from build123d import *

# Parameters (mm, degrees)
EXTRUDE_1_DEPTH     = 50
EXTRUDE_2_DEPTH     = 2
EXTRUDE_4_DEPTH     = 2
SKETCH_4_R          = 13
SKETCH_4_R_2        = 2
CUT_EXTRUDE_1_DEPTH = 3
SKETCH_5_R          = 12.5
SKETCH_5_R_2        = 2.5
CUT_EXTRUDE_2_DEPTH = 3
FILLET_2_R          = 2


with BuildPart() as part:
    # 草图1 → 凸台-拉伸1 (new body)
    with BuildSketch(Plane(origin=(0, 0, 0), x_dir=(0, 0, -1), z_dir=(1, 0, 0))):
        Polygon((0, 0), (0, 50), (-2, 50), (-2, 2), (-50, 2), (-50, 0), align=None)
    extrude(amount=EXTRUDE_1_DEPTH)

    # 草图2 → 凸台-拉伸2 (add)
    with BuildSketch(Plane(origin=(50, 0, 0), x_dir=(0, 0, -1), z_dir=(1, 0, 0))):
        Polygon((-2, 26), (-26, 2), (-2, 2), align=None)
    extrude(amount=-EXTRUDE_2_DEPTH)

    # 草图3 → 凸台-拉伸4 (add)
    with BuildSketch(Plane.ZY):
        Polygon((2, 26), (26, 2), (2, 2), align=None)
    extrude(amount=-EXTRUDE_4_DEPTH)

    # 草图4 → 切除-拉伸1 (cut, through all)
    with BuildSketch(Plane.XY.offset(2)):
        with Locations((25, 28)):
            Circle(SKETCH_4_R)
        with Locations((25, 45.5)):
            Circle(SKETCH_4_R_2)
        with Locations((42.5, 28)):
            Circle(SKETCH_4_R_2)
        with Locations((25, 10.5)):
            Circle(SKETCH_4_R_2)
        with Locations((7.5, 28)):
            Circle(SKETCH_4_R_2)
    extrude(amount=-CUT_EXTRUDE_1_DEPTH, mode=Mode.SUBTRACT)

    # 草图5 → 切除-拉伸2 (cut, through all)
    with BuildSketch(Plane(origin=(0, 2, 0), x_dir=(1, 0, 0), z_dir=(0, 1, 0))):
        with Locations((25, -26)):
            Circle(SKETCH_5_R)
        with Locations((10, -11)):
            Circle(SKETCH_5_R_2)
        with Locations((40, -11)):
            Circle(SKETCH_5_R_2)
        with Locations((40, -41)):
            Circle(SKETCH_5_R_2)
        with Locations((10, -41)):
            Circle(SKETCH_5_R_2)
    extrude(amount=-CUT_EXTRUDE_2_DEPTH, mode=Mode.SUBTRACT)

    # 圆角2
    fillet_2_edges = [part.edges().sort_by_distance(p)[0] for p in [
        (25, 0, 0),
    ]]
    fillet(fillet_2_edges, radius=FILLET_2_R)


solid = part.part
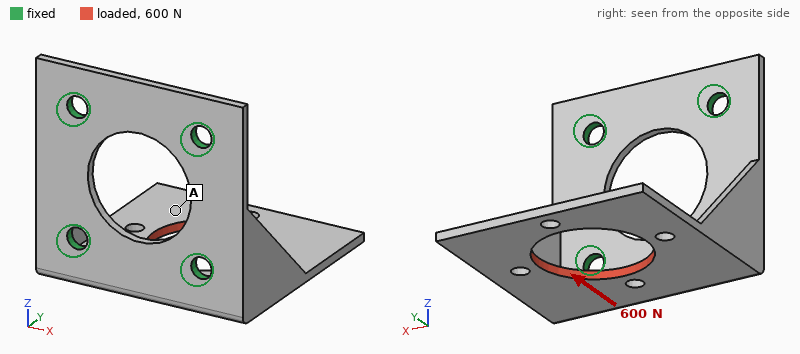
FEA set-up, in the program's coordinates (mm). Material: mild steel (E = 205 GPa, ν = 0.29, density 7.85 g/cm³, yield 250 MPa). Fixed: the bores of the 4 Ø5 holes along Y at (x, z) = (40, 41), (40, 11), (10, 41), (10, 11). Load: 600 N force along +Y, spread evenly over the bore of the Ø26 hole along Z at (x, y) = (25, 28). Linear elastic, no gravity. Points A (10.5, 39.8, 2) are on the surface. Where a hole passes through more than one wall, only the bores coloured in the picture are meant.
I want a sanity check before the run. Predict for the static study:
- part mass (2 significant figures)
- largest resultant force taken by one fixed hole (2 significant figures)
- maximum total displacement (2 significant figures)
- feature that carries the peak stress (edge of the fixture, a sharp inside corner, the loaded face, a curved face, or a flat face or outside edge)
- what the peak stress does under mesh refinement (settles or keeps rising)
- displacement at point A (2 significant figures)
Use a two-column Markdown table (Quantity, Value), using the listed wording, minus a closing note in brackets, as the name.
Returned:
| Quantity | Value |
|---|---|
| part mass | 68 g |
| largest resultant force taken by one fixed hole | 350 N |
| maximum total displacement | 61 µm |
| feature that carries the peak stress | edge of the fixture |
| what the peak stress does under mesh refinement | keeps rising |
| displacement at point A | 47 µm |
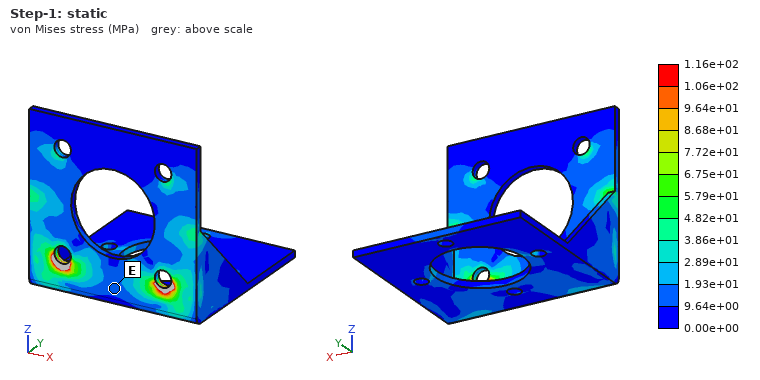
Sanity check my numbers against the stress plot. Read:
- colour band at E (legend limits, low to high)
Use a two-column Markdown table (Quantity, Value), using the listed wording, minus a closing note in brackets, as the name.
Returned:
| Quantity | Value |
|---|---|
| colour band at E | 9.64e+00 to 1.93e+01 MPa |
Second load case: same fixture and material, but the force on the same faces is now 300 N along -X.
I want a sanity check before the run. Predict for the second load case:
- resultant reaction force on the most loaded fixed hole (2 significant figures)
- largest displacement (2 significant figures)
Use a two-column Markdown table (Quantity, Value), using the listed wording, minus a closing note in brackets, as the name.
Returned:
| Quantity | Value |
|---|---|
| resultant reaction force on the most loaded fixed hole | 310 N |
| largest displacement | 48 µm |
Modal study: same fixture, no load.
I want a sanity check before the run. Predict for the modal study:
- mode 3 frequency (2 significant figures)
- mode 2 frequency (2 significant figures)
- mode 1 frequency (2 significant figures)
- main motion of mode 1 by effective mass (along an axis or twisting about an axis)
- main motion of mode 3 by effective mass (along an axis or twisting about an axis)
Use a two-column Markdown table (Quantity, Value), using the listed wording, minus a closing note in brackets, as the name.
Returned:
| Quantity | Value |
|---|---|
| mode 3 frequency | 3600 Hz |
| mode 2 frequency | 2200 Hz |
| mode 1 frequency | 1100 Hz |
| main motion of mode 1 by effective mass | along Z |
| main motion of mode 3 by effective mass | along X |
